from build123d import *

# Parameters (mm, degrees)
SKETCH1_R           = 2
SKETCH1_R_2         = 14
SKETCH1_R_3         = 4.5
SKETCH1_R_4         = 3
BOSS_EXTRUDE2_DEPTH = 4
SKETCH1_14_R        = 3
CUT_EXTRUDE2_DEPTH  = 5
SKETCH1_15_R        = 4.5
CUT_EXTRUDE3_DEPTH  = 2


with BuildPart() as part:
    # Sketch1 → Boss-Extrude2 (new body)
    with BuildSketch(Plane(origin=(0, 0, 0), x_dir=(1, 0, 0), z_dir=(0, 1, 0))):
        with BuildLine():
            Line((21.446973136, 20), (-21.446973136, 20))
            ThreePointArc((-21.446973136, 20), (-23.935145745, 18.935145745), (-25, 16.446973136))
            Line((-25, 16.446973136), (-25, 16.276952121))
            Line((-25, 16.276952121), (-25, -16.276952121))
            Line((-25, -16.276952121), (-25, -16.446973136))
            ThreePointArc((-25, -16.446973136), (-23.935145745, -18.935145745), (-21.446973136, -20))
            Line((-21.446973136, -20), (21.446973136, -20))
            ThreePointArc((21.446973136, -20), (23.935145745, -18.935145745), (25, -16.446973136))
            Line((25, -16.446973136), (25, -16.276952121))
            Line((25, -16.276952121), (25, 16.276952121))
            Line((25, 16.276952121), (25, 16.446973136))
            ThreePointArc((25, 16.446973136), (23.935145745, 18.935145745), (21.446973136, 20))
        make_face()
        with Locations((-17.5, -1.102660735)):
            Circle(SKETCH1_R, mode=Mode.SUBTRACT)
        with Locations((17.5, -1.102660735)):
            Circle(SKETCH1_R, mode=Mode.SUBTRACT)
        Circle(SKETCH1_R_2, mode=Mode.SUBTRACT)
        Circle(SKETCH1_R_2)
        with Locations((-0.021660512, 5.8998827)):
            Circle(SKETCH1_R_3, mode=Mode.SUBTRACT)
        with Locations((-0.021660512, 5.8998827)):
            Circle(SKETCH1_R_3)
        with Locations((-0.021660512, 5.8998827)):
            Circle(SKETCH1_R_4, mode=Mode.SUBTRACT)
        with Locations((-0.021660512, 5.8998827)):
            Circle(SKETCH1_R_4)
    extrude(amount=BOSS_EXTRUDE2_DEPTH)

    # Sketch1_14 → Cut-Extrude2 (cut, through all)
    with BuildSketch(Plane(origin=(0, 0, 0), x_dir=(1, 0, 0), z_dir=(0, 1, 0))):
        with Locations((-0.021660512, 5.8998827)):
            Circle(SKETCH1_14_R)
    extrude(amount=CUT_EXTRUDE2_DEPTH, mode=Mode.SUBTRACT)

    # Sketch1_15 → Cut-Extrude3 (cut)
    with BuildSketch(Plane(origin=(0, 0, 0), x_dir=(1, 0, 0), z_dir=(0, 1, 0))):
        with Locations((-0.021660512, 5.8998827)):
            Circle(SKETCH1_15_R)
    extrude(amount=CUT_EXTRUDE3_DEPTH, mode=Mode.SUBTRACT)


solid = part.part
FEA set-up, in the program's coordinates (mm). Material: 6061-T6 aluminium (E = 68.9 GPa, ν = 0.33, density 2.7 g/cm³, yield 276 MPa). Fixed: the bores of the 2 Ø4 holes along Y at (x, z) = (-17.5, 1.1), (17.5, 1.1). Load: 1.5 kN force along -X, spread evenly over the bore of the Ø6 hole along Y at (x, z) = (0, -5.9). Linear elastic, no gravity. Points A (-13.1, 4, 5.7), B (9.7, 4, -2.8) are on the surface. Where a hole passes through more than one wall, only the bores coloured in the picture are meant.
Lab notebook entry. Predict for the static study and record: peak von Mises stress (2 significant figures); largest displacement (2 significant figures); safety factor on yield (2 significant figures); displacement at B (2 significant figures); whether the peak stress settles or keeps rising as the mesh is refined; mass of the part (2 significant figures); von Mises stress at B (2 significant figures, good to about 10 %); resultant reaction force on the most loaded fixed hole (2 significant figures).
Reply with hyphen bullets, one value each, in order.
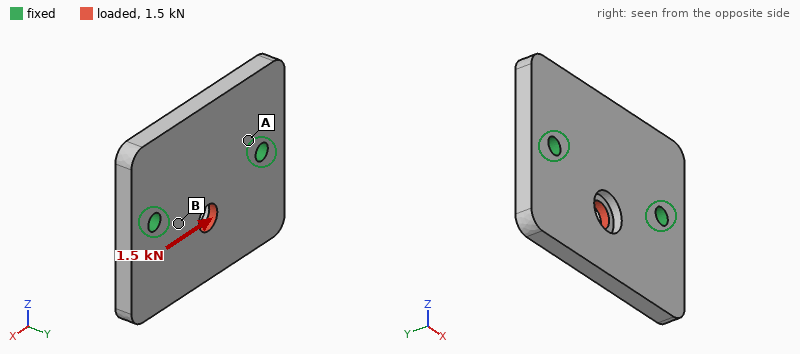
- 71 MPa
- 7.0 µm
- 3.9
- 2.3 µm
- settles
- 21 g
- 23 MPa
- 800 N
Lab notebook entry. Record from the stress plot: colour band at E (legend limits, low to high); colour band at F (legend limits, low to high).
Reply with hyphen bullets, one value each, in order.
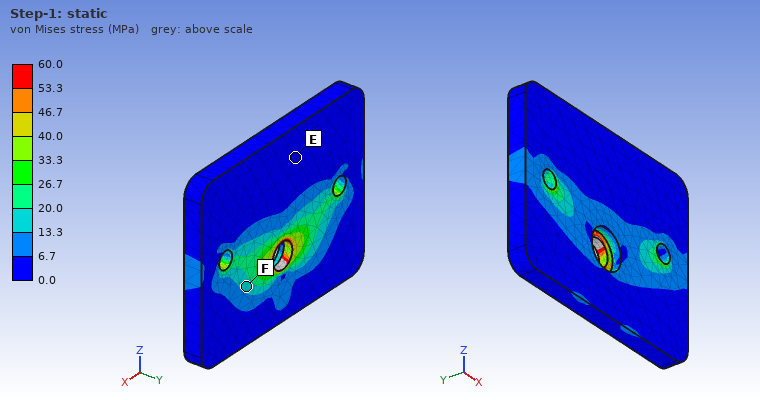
- 0.0 to 6.7 MPa
- 13.3 to 20.0 MPa
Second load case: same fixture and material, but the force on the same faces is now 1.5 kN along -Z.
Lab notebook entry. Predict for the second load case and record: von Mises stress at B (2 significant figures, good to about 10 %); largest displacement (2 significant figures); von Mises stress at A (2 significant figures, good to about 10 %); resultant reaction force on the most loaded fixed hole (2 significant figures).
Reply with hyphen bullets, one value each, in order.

- 18 MPa
- 18 µm
- 15 MPa
- 760 N
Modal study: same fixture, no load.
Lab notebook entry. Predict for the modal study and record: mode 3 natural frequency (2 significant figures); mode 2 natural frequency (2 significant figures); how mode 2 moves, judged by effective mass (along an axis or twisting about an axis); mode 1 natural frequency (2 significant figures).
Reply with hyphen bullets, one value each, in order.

- 10000 Hz
- 8100 Hz
- along Y
- 6000 Hz
